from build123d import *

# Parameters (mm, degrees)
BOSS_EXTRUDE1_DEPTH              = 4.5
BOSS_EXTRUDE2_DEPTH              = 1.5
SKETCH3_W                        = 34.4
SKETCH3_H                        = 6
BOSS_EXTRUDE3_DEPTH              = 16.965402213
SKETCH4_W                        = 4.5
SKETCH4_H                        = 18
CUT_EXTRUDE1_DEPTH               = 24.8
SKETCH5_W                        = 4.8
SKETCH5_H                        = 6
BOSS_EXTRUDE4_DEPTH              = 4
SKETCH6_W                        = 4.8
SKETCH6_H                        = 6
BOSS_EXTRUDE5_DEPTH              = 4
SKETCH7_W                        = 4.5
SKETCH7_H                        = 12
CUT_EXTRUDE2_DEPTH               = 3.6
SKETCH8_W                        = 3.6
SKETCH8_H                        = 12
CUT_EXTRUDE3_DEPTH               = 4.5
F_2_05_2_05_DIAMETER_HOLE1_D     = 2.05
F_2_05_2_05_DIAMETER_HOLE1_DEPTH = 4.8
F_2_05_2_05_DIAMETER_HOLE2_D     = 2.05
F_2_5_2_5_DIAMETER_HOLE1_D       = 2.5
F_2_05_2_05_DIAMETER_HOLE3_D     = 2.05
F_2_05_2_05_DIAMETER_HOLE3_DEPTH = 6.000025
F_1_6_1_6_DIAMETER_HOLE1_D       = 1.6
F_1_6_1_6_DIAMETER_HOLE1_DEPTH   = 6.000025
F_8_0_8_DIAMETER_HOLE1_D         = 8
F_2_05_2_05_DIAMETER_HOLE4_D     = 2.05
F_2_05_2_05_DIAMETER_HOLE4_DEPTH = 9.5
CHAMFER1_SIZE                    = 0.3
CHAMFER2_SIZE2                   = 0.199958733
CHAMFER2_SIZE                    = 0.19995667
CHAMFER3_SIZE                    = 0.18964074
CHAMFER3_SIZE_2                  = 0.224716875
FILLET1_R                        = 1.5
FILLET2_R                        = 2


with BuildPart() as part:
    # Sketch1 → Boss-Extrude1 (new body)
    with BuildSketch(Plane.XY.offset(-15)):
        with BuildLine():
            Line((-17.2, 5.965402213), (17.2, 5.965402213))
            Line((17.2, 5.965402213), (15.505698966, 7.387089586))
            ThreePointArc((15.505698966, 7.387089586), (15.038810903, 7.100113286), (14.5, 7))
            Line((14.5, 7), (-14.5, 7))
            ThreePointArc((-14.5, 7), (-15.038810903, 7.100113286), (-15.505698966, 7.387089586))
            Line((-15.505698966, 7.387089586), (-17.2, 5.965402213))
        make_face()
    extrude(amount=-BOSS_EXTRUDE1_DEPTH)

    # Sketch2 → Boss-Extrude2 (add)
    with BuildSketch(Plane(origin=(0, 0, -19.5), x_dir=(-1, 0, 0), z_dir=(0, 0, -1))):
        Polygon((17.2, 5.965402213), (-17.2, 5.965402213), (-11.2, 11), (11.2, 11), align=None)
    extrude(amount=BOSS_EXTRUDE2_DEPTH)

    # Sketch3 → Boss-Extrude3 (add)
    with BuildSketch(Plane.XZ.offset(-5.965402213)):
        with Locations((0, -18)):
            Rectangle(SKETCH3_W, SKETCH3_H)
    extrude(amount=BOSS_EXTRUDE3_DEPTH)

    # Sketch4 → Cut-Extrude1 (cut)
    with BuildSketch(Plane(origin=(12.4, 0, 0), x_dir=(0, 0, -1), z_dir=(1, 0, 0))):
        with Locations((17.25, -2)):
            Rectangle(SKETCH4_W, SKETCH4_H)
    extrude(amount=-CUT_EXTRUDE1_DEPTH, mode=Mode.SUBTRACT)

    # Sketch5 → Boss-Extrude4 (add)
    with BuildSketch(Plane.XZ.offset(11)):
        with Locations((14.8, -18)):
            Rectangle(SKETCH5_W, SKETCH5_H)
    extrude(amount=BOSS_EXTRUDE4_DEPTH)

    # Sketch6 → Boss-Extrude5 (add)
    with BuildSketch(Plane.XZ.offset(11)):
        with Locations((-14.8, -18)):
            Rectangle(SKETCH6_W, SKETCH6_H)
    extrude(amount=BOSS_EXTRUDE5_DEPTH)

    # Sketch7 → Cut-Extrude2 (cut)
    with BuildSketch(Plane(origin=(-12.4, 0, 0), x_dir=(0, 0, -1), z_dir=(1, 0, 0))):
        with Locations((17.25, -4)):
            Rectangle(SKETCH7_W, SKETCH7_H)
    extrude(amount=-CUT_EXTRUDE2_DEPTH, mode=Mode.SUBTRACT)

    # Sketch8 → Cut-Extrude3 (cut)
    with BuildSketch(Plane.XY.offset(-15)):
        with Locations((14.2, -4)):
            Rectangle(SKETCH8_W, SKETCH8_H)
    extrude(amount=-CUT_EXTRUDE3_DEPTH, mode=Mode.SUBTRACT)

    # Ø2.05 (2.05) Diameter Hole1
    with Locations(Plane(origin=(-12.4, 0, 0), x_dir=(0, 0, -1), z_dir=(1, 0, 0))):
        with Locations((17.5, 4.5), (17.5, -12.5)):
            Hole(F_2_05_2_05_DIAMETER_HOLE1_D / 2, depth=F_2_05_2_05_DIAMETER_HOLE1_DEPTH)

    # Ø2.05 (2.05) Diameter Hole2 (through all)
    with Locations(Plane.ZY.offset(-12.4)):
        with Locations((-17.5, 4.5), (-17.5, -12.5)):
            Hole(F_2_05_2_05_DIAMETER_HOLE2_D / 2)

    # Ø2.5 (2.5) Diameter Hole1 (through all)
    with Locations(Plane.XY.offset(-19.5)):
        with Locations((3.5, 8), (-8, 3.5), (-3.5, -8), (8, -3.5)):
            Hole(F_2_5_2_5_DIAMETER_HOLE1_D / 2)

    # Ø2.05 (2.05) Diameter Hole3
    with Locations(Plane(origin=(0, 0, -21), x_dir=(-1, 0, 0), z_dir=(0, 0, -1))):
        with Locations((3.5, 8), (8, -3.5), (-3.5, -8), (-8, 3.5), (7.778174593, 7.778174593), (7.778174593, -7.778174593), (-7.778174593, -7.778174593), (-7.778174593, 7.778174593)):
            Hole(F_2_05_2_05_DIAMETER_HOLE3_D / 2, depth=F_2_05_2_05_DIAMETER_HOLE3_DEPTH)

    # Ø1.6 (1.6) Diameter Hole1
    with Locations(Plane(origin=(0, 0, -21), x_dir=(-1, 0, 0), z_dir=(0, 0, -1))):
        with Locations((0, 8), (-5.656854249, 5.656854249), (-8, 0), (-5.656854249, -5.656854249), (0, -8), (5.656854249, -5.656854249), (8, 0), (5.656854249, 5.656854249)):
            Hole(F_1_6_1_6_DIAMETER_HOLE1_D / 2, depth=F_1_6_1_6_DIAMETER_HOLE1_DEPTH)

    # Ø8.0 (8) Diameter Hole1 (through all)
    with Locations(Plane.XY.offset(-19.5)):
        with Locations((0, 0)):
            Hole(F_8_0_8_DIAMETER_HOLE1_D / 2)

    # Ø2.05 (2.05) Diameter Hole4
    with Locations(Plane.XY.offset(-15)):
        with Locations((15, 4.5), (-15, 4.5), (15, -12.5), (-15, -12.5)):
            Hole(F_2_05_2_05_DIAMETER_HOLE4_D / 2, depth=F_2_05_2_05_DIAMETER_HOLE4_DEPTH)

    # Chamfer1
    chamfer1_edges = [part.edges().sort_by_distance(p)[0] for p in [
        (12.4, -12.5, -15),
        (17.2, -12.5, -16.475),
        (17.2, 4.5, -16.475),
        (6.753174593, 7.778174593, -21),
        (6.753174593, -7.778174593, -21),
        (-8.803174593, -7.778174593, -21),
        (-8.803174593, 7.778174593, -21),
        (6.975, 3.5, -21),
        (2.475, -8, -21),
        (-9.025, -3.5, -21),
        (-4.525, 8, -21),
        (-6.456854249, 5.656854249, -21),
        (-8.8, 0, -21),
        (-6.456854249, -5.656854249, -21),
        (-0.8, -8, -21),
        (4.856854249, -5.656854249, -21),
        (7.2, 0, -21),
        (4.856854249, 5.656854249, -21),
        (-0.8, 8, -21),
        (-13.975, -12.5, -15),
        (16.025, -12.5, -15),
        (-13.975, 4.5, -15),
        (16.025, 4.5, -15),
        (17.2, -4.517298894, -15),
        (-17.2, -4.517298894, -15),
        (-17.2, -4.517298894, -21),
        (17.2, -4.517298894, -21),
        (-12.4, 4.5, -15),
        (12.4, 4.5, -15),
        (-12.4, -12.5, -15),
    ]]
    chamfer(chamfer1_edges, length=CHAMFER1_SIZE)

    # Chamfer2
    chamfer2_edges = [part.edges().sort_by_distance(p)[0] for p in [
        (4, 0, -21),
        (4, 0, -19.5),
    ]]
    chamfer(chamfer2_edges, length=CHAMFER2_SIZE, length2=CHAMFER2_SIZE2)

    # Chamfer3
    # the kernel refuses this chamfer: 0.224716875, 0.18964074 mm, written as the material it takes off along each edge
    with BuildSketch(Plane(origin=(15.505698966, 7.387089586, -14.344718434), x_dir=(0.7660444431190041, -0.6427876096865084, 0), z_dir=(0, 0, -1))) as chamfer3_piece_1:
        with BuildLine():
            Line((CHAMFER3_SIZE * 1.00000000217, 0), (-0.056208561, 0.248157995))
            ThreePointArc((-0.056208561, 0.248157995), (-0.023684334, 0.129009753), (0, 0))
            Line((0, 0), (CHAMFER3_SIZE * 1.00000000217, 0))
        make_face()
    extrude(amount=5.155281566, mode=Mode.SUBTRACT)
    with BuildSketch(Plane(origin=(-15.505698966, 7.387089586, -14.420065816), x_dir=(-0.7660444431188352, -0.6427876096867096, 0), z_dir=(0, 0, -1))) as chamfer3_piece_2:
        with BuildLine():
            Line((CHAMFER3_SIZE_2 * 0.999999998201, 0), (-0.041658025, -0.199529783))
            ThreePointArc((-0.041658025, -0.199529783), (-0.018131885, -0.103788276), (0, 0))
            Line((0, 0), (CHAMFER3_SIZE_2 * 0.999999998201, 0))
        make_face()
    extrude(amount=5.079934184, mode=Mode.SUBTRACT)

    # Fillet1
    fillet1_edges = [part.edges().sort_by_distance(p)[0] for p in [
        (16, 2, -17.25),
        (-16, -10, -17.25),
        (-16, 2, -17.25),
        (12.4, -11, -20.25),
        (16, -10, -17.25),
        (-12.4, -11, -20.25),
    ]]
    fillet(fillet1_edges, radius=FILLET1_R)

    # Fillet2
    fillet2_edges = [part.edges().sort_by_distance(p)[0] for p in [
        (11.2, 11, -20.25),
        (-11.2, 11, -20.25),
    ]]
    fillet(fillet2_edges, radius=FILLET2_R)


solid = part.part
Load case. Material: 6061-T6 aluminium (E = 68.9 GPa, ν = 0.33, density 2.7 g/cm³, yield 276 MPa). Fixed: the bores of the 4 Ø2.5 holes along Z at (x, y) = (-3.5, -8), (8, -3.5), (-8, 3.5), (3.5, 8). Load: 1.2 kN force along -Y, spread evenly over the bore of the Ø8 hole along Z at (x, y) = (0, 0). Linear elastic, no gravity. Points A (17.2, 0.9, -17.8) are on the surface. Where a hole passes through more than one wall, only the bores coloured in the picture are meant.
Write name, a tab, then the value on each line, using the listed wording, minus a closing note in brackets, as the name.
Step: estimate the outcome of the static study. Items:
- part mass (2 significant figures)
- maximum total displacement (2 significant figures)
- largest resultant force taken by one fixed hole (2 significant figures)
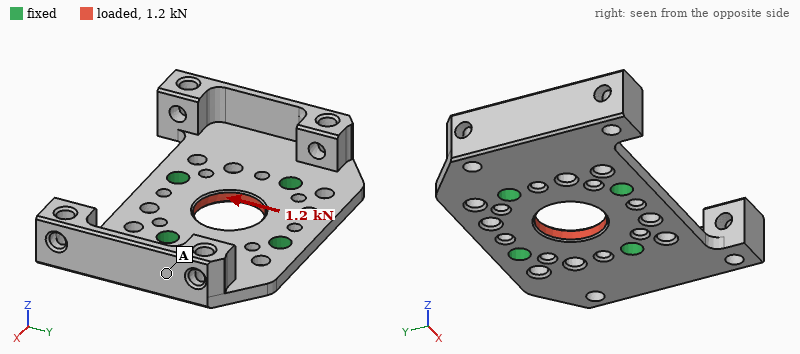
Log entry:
part mass	3.8 g
maximum total displacement	4.9 µm
largest resultant force taken by one fixed hole	350 N
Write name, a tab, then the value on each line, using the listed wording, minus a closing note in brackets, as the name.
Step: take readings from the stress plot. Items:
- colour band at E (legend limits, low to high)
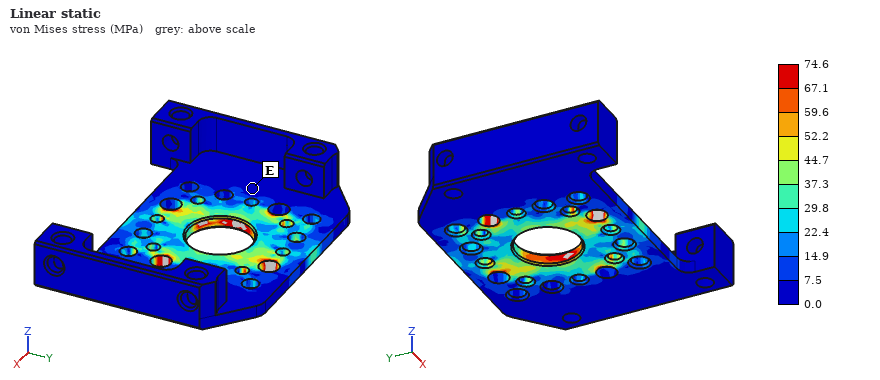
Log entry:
colour band at E	0.0 to 7.5 MPa
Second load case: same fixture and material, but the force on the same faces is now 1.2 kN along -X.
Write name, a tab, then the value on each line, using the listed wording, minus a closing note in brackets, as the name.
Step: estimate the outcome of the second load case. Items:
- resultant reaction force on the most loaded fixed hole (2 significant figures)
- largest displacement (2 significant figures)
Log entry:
resultant reaction force on the most loaded fixed hole	360 N
largest displacement	4.4 µm
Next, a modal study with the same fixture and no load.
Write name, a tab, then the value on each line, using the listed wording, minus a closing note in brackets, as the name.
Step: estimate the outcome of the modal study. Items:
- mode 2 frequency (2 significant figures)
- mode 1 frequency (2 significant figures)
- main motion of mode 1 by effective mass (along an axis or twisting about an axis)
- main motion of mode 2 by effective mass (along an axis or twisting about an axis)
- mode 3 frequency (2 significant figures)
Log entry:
mode 2 frequency	6700 Hz
mode 1 frequency	4900 Hz
main motion of mode 1 by effective mass	along Z
main motion of mode 2 by effective mass	along Z
mode 3 frequency	7600 Hz
